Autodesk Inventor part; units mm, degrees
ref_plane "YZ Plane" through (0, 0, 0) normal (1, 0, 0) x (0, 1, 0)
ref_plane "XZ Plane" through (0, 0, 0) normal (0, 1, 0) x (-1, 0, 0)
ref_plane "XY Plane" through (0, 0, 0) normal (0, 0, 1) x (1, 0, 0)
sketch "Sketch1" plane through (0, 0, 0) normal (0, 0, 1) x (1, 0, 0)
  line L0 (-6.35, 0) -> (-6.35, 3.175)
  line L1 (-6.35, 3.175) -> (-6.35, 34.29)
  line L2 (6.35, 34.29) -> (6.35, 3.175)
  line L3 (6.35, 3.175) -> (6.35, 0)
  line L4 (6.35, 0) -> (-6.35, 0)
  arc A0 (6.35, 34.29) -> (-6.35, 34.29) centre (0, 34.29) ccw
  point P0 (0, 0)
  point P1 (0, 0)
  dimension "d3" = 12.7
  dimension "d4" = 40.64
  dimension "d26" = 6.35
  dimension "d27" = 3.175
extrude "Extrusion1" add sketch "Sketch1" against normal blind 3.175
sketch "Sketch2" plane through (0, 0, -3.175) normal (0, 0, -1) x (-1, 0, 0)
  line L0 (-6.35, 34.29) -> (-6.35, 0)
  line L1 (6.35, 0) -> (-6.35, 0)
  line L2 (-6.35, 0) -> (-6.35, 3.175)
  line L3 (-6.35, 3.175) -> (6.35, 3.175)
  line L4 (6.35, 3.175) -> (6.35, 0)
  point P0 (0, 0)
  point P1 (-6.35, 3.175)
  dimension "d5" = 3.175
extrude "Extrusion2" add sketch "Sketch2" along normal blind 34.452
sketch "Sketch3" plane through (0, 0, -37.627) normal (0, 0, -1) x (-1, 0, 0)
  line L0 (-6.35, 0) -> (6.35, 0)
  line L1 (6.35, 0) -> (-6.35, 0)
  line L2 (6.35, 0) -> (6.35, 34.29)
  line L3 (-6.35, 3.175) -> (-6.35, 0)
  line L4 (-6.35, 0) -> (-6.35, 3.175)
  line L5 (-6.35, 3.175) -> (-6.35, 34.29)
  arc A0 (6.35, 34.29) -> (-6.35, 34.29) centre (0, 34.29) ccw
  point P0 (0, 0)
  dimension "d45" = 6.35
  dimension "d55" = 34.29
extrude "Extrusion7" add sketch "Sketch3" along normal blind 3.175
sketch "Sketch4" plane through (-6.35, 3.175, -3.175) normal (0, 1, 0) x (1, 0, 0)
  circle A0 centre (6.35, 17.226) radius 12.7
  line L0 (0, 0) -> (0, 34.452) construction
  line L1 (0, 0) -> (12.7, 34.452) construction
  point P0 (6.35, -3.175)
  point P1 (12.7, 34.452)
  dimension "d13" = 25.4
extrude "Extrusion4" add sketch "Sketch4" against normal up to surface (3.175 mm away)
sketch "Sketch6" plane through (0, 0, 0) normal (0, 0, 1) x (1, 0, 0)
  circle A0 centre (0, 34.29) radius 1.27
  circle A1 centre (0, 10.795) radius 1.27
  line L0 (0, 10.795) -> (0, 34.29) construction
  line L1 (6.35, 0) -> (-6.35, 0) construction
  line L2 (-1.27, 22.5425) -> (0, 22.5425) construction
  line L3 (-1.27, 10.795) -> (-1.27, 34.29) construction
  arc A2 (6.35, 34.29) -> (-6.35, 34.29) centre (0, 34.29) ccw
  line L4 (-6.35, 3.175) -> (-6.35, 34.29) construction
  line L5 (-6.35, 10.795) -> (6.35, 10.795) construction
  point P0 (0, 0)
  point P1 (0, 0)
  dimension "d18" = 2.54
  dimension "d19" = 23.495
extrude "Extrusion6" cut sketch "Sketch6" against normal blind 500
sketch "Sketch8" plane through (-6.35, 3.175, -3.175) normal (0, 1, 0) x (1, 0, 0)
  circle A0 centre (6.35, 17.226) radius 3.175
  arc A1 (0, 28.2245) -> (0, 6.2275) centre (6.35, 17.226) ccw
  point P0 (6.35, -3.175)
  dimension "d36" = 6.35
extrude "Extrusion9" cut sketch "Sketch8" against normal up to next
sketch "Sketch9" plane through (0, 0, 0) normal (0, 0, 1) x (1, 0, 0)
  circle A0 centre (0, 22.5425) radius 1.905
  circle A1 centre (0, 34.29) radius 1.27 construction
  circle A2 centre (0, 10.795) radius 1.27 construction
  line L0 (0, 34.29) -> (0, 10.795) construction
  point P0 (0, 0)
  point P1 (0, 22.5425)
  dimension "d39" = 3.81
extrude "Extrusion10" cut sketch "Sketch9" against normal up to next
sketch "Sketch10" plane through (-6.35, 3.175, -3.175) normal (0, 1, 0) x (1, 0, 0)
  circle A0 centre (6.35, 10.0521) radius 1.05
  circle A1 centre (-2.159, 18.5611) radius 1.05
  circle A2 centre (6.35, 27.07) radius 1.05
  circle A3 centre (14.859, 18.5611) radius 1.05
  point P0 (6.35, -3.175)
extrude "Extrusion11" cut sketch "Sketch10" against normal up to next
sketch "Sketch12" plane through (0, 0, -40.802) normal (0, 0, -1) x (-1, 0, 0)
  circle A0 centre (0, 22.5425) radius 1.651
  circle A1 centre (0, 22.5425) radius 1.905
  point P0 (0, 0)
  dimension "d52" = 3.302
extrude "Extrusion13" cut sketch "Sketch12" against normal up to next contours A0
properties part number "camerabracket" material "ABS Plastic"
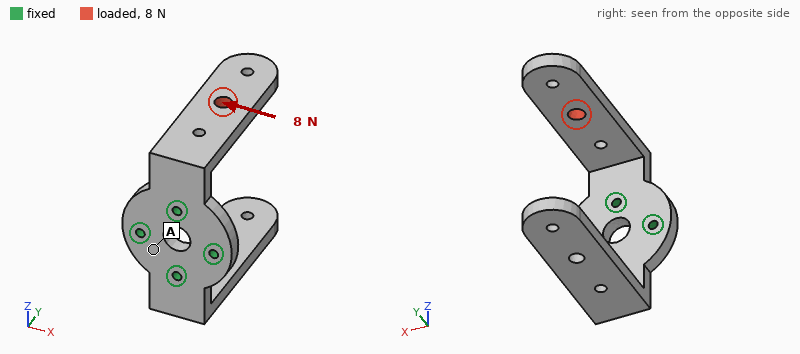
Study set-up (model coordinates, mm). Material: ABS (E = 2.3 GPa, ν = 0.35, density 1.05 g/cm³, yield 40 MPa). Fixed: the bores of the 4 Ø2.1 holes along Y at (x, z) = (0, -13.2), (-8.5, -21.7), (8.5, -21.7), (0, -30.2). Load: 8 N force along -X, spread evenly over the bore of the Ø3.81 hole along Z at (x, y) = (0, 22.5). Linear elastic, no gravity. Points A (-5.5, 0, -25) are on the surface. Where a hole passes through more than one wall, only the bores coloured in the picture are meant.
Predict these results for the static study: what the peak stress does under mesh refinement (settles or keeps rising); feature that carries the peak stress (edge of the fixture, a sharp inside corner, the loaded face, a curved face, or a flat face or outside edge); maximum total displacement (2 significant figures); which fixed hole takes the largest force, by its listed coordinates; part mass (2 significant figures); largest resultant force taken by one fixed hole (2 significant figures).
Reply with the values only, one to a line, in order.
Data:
keeps rising
edge of the fixture
0.64 mm
(0, -13.2)
5.2 g
7.0 N
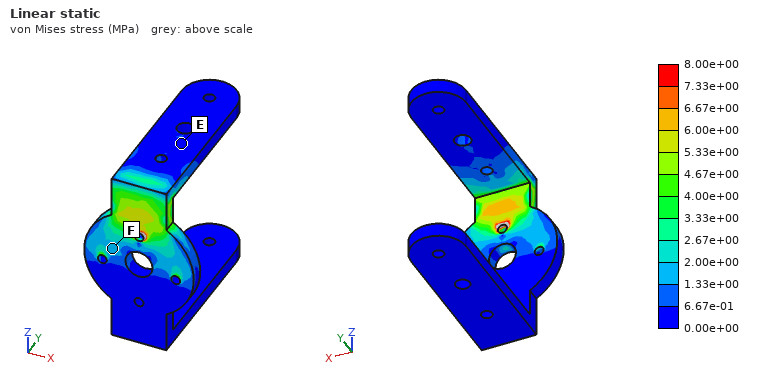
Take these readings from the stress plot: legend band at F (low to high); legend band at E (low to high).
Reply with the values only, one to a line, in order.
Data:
1.33e+00 to 2.00e+00 MPa
0.00e+00 to 6.67e-01 MPa
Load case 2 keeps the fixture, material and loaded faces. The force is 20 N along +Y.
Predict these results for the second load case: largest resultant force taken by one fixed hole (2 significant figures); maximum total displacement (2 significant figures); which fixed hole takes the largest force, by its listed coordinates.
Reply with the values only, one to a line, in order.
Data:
30 N
0.66 mm
(0, -13.2)
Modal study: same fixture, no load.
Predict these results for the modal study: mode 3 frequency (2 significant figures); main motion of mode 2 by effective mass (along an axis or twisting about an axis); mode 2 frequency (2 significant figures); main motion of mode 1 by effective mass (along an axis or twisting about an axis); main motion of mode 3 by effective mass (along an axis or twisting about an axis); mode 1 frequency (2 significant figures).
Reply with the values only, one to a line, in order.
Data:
590 Hz
along Z
400 Hz
along Z
along X
370 Hz
